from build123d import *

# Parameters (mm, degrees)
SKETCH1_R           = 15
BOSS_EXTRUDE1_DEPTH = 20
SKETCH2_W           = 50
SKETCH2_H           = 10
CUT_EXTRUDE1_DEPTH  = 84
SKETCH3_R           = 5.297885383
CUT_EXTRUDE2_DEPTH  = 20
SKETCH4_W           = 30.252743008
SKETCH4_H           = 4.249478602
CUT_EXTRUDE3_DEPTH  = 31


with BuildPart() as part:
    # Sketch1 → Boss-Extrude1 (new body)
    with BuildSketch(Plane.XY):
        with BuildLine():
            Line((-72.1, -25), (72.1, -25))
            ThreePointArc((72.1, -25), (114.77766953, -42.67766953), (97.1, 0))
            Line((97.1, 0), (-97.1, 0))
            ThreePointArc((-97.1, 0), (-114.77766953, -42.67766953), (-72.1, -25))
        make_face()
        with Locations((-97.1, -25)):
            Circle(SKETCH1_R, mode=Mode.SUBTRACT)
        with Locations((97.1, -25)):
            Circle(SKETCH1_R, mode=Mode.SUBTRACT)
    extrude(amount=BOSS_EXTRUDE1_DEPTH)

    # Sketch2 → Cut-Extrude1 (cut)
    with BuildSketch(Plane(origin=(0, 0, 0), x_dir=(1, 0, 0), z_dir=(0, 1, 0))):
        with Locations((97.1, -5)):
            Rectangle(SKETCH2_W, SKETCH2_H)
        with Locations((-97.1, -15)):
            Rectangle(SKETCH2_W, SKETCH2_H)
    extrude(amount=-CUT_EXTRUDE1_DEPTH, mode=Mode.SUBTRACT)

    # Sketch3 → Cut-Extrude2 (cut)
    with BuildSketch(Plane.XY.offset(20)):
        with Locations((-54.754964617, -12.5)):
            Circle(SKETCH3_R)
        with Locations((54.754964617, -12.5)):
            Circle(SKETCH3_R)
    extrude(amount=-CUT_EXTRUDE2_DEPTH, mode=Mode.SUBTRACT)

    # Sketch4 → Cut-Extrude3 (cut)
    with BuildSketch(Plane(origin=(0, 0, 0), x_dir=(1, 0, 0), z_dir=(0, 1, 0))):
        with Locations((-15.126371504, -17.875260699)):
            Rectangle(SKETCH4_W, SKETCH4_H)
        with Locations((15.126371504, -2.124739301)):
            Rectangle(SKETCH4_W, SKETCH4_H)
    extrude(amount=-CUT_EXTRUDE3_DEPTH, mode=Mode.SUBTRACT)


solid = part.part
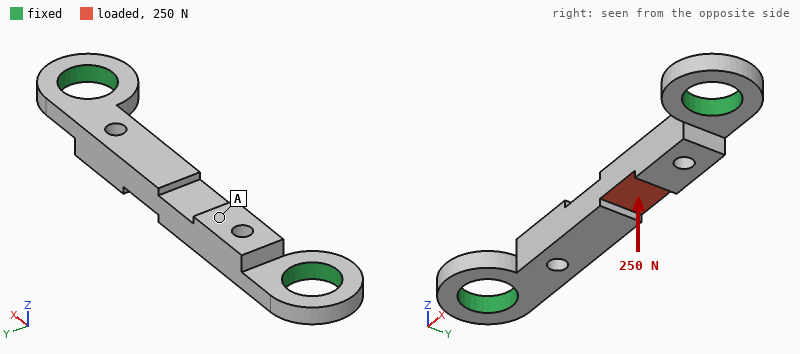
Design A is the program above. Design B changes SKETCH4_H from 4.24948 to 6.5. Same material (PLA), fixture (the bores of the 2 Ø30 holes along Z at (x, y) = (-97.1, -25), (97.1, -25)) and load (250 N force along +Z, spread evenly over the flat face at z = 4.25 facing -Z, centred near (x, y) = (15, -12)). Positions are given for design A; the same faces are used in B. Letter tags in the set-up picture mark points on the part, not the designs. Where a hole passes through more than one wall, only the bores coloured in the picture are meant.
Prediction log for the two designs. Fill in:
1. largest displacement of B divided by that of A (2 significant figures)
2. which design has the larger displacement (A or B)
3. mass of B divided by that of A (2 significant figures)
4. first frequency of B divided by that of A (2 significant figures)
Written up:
1.2
B
0.98
0.94
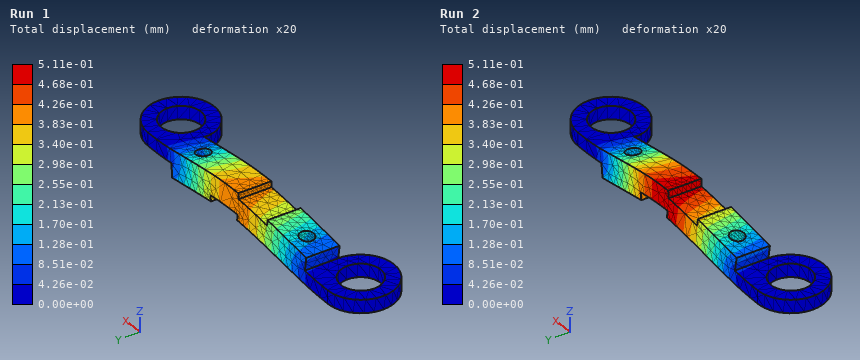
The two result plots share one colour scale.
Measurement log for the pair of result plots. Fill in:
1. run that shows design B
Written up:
Run 2
